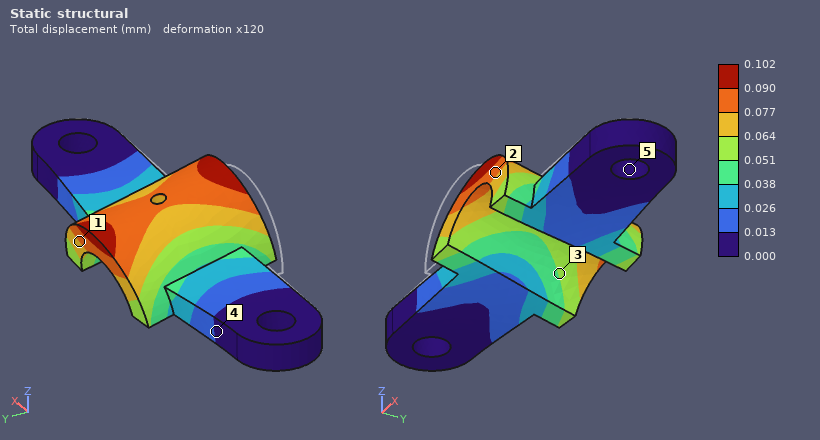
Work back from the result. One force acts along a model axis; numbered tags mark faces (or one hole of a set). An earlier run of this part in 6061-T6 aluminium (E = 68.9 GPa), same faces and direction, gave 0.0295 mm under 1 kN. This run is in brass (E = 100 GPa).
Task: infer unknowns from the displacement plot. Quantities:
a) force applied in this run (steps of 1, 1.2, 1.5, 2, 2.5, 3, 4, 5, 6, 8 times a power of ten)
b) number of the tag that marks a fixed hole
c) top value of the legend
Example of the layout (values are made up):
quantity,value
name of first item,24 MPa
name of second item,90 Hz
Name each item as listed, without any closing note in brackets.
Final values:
quantity,value
force applied in this run,5 kN
number of the tag that marks a fixed hole,5
top value of the legend,0.102 mm
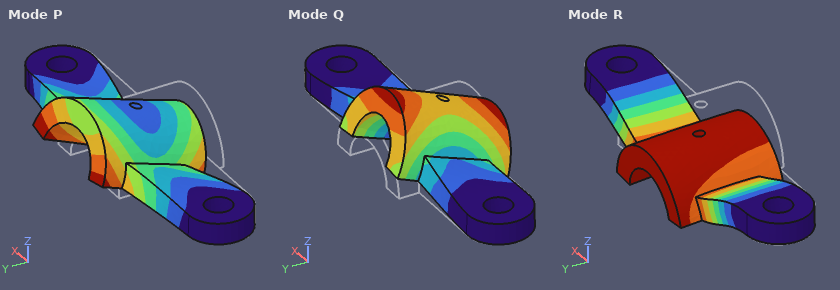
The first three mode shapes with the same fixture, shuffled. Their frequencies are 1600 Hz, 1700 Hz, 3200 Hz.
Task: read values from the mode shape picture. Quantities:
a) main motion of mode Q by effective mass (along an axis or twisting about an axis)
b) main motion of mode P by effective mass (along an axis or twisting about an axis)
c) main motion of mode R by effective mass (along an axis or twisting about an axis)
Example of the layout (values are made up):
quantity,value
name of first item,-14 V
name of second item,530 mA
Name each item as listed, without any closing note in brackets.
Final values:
quantity,value
main motion of mode Q by effective mass,along Y
main motion of mode P by effective mass,along Y
main motion of mode R by effective mass,along Z
